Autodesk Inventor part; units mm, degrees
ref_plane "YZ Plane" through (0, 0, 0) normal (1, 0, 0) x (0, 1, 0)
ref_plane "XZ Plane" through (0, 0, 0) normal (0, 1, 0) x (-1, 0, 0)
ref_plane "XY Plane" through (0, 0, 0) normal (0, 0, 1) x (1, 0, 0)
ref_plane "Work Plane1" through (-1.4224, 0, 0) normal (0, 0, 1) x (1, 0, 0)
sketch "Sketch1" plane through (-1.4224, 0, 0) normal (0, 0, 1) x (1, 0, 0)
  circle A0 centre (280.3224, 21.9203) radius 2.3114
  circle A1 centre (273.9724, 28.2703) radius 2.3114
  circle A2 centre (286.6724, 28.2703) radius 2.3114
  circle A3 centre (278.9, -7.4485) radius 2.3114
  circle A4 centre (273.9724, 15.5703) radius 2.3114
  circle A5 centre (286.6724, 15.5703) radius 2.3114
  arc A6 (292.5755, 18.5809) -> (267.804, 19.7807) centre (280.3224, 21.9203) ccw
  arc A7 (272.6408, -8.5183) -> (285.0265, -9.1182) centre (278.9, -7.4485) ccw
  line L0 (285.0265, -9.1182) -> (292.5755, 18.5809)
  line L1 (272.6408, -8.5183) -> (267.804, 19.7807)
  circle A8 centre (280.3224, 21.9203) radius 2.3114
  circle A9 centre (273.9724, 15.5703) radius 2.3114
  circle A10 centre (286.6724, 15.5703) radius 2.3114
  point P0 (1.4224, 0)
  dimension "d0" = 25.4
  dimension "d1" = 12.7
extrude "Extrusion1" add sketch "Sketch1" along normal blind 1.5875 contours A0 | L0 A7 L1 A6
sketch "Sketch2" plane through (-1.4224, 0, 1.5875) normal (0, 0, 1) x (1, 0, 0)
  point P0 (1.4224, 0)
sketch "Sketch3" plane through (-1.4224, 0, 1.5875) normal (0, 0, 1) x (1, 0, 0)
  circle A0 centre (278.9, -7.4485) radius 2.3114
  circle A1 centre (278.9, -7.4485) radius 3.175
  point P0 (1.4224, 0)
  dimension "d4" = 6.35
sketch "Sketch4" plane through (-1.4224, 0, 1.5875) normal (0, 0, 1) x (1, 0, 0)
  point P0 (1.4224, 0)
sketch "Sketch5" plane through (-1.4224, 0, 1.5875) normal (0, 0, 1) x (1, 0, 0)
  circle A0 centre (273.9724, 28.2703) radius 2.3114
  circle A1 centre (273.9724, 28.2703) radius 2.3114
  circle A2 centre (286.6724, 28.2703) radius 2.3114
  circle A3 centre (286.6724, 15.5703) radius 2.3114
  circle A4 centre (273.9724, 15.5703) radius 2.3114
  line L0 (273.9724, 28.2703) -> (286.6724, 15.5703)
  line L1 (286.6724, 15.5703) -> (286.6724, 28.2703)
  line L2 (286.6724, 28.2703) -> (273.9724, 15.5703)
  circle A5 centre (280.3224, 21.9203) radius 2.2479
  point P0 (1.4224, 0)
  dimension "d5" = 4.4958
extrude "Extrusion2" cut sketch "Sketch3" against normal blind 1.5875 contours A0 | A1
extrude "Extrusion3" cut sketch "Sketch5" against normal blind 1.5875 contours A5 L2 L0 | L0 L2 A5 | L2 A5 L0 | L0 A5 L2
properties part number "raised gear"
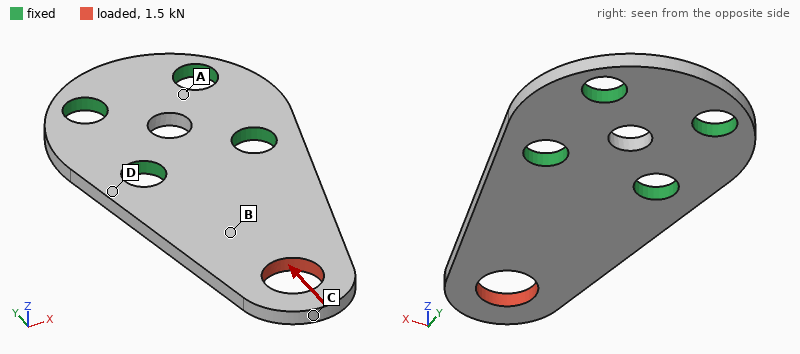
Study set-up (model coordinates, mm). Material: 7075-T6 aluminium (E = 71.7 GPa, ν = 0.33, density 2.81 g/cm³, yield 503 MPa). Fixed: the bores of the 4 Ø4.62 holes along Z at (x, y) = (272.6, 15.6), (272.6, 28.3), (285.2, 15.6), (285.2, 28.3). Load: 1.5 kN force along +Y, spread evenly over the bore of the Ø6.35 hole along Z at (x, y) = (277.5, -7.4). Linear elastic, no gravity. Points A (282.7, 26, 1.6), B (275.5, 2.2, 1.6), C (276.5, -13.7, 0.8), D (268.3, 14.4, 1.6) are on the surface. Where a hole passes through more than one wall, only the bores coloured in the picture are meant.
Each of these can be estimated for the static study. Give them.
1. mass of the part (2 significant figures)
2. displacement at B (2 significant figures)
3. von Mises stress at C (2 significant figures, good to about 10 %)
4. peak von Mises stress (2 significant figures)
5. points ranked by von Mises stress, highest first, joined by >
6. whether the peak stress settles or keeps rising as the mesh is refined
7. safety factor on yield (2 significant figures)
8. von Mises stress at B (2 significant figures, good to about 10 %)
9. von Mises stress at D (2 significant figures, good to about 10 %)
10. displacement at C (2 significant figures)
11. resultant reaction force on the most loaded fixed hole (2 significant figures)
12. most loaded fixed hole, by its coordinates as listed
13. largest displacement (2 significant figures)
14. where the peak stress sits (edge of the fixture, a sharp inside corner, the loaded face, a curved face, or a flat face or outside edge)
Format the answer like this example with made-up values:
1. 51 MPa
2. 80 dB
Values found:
1. 3.5 g
2. 9.5 µm
3. 86 MPa
4. 200 MPa
5. C > B > D > A
6. settles
7. 2.5
8. 55 MPa
9. 29 MPa
10. 29 µm
11. 850 N
12. (272.6, 15.6)
13. 30 µm
14. the loaded face
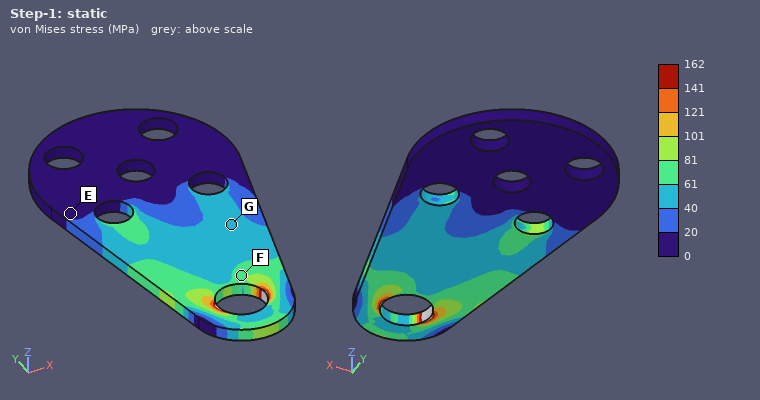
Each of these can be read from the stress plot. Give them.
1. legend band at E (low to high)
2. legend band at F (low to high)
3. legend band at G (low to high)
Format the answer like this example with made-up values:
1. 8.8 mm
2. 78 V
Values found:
1. 0 to 20 MPa
2. 61 to 81 MPa
3. 40 to 61 MPa
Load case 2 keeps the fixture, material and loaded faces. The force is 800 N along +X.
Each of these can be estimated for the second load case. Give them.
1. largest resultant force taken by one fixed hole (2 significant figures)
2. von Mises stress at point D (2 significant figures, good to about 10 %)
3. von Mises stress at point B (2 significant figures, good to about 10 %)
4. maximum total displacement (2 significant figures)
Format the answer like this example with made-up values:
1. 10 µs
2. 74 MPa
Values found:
1. 1.2 kN
2. 72 MPa
3. 61 MPa
4. 96 µm
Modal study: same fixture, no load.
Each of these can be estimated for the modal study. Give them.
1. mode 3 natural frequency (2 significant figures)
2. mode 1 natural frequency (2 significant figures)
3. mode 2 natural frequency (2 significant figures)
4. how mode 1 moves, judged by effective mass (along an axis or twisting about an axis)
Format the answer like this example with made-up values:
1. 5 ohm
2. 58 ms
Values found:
1. 11 kHz
2. 2500 Hz
3. 8900 Hz
4. along Z
